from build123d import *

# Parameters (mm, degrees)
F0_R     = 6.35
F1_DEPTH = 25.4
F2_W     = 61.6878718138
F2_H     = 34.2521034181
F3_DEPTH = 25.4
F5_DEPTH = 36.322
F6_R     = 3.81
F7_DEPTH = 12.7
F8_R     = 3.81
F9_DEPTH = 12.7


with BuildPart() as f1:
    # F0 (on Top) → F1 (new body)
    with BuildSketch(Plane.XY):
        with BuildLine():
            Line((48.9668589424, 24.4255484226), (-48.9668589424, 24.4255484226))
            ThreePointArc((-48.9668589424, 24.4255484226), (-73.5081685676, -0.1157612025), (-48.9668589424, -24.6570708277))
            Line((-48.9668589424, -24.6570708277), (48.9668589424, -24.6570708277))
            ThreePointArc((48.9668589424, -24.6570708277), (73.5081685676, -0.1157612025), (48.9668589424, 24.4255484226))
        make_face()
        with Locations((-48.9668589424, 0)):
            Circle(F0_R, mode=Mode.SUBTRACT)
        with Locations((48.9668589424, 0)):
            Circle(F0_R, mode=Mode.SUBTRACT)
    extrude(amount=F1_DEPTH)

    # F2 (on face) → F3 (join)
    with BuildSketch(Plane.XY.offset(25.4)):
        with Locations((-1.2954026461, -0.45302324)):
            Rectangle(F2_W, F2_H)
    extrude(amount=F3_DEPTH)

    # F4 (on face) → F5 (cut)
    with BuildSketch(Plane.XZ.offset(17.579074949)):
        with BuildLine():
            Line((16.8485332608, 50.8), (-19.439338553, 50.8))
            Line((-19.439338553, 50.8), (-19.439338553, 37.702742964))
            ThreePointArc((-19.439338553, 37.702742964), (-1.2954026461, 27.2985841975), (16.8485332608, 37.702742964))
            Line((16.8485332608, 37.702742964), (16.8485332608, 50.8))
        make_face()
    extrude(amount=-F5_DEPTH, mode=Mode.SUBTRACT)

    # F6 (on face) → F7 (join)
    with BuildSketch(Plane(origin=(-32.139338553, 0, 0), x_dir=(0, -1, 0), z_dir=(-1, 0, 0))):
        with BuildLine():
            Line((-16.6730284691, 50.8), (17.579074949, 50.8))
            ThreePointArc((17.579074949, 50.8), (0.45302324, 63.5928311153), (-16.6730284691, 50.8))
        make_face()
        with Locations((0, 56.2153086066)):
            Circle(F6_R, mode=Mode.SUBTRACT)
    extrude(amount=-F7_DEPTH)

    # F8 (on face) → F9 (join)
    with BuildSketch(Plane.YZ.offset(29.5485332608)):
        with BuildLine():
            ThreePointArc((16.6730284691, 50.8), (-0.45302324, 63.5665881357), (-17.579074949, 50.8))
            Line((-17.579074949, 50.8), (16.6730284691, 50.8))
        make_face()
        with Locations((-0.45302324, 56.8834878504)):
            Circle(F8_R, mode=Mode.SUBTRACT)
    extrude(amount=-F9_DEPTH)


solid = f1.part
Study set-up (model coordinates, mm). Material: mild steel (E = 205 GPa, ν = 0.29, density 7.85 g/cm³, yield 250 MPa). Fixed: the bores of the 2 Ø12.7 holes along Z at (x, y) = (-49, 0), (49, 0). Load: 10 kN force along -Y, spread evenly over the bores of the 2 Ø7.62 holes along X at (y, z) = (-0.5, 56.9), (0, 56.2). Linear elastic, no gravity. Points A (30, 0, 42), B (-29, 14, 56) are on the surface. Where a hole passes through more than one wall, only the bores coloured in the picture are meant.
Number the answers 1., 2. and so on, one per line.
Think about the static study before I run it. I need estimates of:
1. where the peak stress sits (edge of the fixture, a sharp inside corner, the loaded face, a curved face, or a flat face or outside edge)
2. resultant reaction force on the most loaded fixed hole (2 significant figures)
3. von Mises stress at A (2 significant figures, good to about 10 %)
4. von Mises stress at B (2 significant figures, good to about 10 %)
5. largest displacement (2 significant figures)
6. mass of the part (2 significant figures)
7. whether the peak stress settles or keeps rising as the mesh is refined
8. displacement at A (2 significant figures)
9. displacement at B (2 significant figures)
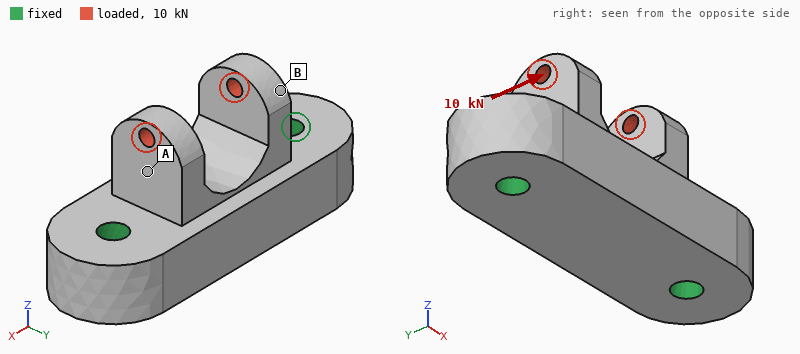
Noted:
1. edge of the fixture
2. 5.2 kN
3. 29 MPa
4. 11 MPa
5. 35 µm
6. 1.6 kg
7. keeps rising
8. 17 µm
9. 29 µm
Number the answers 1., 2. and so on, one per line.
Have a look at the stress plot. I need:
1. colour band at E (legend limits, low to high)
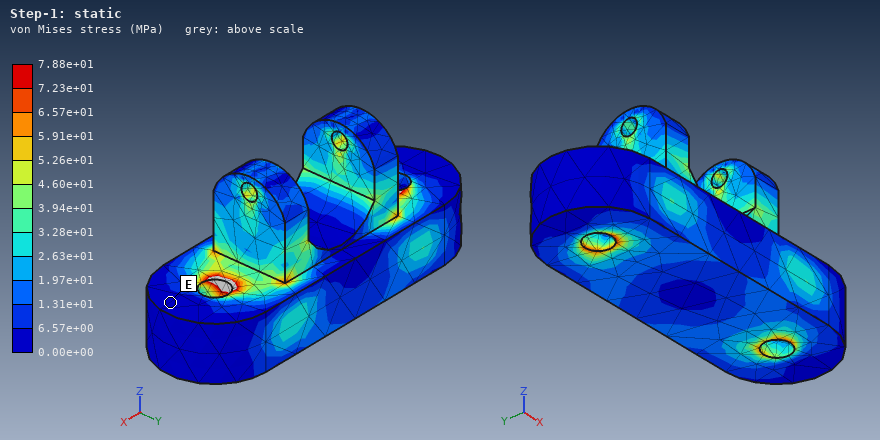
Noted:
1. 0.00e+00 to 6.57e+00 MPa
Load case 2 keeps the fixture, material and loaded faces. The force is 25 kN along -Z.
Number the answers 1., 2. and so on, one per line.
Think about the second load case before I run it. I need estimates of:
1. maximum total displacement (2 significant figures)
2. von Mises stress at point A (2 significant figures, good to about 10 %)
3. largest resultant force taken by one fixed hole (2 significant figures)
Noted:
1. 16 µm
2. 40 MPa
3. 13 kN
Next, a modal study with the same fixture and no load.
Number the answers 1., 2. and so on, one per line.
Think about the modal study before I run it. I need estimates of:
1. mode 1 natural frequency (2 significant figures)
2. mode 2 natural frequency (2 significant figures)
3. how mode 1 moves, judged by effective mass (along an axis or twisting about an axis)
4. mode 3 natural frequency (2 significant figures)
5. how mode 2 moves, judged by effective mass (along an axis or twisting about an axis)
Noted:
1. 7300 Hz
2. 7900 Hz
3. along Y
4. 9400 Hz
5. along Z
